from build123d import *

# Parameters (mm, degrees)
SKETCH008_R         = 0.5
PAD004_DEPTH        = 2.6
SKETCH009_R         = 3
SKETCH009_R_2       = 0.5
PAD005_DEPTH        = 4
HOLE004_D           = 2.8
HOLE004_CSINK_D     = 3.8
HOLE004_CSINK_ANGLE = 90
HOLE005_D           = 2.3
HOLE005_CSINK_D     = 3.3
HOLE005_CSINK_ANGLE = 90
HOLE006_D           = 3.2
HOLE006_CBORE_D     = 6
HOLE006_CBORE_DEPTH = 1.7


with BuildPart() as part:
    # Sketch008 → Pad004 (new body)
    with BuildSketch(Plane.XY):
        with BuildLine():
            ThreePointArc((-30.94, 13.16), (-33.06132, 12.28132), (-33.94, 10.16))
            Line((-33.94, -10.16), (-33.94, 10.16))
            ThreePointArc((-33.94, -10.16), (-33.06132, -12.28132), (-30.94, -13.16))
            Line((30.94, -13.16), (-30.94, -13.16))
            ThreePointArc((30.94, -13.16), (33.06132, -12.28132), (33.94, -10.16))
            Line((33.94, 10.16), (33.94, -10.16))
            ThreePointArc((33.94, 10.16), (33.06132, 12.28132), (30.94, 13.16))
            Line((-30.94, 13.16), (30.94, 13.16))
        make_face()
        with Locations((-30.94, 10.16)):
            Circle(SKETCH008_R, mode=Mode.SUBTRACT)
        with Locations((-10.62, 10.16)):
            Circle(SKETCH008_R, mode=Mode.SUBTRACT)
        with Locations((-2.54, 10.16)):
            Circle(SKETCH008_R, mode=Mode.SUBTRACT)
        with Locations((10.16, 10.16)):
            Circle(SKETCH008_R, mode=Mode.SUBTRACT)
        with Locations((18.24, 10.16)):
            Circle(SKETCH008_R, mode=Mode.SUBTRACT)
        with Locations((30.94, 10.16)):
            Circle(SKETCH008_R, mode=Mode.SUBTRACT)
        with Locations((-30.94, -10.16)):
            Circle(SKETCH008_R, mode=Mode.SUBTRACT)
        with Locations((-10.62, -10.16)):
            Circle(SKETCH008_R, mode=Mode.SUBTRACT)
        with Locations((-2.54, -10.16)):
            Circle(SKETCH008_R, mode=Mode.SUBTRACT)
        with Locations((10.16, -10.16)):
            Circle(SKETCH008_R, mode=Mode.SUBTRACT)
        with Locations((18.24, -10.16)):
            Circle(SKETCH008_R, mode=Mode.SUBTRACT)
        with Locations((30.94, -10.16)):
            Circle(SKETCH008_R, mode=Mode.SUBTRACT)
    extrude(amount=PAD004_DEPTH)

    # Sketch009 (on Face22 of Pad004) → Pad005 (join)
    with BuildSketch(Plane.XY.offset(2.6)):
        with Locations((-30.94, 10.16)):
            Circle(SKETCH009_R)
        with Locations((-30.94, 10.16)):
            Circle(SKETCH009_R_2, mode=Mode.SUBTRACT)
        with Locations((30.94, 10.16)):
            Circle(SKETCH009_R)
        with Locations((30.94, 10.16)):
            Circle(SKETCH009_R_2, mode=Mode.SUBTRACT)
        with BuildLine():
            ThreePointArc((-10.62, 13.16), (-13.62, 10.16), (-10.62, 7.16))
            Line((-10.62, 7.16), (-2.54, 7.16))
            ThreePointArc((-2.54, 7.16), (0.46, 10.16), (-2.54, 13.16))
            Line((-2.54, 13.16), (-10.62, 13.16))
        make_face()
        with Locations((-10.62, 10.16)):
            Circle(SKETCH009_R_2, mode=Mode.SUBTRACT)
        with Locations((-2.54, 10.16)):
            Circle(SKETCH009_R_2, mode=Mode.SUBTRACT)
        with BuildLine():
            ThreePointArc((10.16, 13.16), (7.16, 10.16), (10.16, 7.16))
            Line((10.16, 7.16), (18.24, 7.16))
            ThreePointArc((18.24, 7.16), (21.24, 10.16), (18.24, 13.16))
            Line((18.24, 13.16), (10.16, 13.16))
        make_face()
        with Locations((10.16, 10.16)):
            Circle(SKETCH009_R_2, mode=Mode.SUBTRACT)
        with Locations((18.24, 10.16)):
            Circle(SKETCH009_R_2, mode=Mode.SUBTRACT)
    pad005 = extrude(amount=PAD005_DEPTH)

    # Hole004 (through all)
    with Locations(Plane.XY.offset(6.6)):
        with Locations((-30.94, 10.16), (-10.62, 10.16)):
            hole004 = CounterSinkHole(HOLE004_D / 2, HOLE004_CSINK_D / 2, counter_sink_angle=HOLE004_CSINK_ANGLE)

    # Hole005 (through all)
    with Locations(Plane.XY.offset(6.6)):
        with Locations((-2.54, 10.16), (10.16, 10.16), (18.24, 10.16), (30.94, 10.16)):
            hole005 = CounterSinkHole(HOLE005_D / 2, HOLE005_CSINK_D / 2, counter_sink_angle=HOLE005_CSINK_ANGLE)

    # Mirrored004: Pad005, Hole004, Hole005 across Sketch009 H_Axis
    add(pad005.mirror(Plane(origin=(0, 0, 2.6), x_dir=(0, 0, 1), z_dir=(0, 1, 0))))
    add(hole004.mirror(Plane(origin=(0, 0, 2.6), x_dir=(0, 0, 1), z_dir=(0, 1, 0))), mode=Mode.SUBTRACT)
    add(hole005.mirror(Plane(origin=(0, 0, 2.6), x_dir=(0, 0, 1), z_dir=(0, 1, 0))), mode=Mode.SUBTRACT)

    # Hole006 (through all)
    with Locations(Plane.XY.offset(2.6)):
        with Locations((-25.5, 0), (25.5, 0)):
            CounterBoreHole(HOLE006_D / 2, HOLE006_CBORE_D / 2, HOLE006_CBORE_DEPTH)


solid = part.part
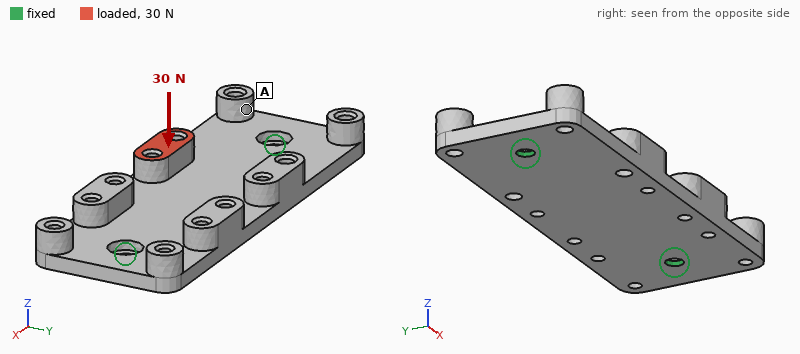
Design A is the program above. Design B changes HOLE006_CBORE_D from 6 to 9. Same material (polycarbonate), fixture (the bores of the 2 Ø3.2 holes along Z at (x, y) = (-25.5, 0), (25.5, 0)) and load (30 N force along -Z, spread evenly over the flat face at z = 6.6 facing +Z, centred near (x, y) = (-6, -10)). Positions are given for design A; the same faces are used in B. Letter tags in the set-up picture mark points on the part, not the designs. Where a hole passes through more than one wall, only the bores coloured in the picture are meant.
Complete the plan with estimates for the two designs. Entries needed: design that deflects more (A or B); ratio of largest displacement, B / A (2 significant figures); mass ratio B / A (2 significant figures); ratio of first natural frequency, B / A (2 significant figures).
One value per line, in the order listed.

B
1.3
0.98
0.82
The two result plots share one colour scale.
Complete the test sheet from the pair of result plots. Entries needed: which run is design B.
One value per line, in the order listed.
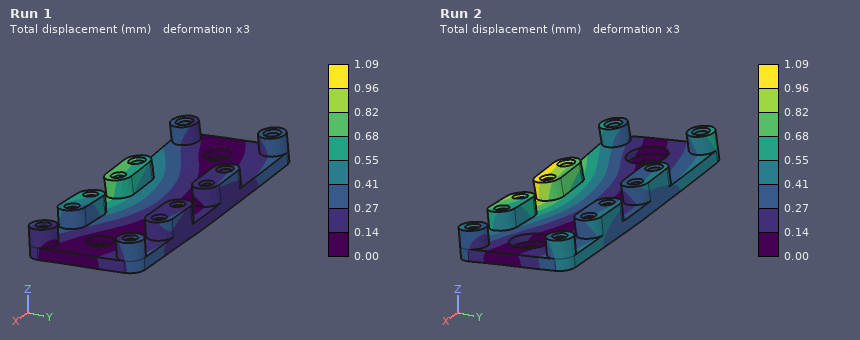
Run 2
